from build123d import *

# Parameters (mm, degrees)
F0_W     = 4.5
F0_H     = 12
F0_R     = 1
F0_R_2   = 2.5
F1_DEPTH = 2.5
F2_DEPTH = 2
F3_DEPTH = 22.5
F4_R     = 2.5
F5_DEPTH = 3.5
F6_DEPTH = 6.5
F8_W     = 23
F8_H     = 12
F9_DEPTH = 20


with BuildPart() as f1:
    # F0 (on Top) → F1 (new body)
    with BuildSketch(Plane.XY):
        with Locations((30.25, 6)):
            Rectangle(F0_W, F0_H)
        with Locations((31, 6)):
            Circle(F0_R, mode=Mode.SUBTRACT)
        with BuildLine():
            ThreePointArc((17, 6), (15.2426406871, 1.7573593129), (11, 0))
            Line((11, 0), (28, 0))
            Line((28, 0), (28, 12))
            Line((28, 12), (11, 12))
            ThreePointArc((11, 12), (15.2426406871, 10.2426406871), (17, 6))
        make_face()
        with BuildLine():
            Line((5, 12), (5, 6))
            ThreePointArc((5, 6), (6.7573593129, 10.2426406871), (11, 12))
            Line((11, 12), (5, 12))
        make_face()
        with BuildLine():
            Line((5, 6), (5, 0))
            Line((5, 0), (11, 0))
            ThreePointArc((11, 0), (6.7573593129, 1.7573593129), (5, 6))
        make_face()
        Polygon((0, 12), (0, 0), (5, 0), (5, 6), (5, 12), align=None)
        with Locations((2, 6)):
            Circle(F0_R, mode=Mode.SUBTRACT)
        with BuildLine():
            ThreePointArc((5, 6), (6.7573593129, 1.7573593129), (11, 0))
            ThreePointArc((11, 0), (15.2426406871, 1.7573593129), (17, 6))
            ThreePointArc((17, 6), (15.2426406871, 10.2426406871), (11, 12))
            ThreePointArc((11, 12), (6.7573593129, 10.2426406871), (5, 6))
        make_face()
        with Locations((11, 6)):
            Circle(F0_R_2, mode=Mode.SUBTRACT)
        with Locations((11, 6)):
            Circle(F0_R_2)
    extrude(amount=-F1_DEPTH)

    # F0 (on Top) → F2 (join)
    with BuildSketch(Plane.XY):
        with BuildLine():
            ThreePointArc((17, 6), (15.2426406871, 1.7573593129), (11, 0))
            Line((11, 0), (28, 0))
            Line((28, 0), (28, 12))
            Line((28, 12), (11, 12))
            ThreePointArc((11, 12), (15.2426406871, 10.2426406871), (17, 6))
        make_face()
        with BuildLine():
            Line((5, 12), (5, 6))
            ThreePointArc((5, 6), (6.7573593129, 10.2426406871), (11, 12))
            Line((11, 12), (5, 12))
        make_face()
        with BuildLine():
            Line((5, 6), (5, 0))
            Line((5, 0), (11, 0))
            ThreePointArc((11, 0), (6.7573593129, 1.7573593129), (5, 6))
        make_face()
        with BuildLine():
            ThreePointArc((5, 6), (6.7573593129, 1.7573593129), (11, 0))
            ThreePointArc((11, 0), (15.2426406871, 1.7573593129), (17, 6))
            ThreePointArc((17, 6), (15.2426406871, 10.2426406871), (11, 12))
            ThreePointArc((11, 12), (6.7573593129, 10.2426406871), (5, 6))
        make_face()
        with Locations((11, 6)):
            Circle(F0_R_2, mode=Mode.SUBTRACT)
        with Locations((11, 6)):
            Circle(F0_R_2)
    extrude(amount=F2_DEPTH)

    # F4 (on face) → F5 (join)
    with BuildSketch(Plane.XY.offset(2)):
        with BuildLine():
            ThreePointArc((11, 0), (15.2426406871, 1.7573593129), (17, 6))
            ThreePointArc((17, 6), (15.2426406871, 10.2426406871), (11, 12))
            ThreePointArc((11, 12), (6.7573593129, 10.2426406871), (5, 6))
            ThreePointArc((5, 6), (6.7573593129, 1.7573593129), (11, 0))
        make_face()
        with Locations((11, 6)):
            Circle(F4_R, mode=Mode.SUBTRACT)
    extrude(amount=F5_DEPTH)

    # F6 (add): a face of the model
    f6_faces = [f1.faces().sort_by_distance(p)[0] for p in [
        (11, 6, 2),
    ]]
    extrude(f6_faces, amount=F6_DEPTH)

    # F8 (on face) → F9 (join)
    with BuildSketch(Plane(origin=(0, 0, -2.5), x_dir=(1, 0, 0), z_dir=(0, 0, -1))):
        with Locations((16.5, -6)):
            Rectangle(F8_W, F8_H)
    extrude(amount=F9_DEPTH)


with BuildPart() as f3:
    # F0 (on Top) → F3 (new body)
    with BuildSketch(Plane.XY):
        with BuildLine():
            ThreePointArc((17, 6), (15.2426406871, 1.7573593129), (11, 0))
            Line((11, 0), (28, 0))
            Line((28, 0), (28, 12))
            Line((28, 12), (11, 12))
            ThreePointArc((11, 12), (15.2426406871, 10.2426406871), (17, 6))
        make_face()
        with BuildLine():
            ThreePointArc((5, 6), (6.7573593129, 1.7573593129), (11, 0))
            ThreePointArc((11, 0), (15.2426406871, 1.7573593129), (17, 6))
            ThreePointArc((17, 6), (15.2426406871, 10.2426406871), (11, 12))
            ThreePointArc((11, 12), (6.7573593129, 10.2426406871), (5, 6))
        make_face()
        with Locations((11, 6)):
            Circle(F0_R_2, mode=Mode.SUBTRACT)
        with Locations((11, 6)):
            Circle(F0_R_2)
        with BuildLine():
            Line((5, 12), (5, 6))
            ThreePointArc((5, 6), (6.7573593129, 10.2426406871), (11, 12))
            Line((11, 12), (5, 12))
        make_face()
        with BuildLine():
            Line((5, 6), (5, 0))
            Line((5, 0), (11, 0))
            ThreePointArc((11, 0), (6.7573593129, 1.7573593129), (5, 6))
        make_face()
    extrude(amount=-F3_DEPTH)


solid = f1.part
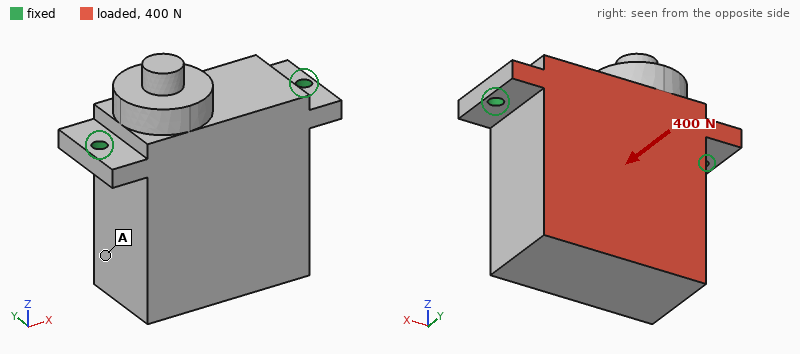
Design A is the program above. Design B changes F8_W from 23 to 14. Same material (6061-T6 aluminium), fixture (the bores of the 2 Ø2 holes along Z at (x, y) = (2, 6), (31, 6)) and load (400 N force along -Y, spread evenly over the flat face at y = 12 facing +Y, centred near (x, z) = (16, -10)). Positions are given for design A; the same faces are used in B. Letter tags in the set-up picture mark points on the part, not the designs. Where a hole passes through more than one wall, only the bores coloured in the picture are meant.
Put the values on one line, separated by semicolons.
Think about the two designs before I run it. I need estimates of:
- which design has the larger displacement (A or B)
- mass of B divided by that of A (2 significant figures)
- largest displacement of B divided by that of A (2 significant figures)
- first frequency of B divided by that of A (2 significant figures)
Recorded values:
B; 0.71; 1.2; 1.1
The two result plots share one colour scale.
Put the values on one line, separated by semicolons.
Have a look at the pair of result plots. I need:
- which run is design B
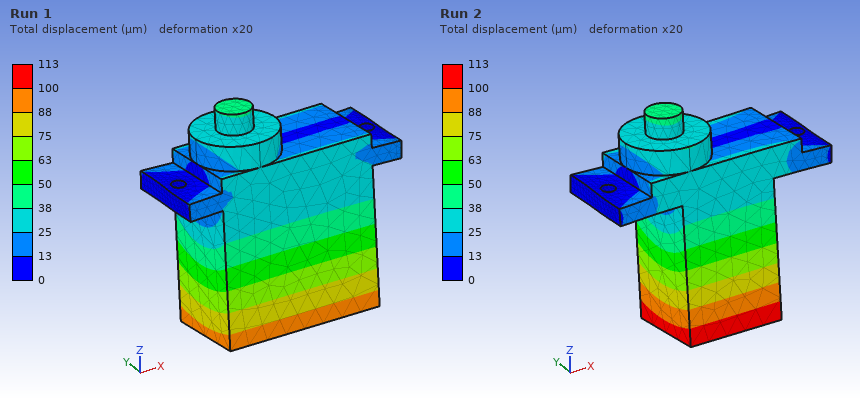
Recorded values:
Run 2
